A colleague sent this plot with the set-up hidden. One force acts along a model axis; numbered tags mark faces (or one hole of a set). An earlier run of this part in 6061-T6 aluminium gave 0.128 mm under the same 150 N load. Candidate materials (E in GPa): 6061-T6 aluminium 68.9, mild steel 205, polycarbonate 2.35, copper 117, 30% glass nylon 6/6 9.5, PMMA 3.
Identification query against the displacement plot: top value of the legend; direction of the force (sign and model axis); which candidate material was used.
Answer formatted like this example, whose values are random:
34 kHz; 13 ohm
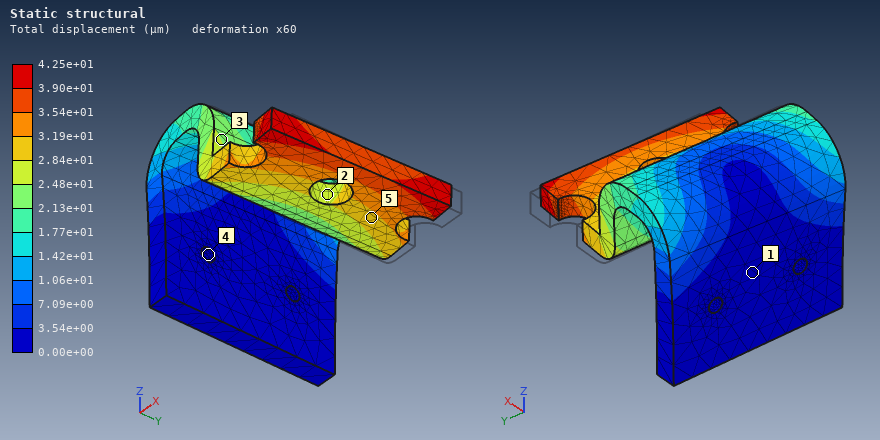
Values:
4.25e+01 µm; -Y; mild steel
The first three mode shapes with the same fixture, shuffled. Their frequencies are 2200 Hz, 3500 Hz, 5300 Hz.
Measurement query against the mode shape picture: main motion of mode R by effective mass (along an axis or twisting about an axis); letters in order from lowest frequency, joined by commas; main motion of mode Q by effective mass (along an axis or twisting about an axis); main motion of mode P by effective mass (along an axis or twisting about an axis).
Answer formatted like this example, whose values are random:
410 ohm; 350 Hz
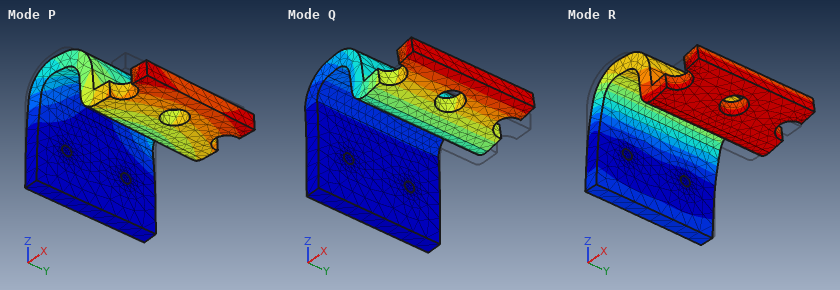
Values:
along X; Q, P, R; along Z; along Y
